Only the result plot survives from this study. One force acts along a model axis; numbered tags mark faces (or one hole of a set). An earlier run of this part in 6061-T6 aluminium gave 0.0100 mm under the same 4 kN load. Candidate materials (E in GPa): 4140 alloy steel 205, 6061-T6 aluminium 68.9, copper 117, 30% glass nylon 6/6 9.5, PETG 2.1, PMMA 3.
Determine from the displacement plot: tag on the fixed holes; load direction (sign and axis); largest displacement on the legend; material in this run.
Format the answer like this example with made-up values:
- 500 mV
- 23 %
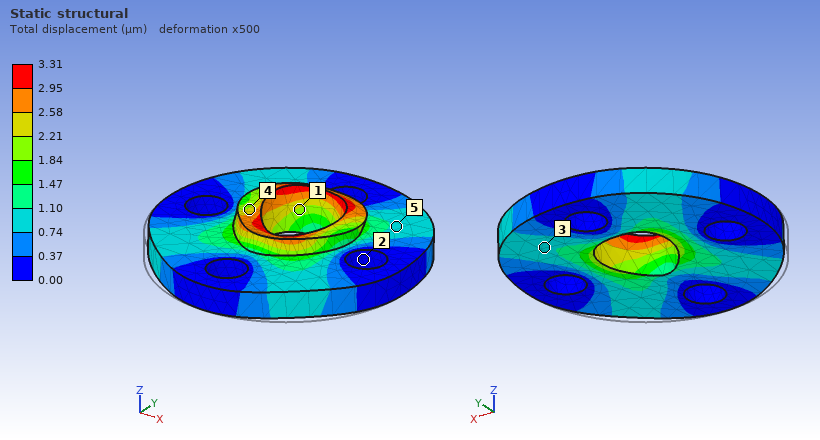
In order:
- 2
- +Y
- 3.31 µm
- 4140 alloy steel
